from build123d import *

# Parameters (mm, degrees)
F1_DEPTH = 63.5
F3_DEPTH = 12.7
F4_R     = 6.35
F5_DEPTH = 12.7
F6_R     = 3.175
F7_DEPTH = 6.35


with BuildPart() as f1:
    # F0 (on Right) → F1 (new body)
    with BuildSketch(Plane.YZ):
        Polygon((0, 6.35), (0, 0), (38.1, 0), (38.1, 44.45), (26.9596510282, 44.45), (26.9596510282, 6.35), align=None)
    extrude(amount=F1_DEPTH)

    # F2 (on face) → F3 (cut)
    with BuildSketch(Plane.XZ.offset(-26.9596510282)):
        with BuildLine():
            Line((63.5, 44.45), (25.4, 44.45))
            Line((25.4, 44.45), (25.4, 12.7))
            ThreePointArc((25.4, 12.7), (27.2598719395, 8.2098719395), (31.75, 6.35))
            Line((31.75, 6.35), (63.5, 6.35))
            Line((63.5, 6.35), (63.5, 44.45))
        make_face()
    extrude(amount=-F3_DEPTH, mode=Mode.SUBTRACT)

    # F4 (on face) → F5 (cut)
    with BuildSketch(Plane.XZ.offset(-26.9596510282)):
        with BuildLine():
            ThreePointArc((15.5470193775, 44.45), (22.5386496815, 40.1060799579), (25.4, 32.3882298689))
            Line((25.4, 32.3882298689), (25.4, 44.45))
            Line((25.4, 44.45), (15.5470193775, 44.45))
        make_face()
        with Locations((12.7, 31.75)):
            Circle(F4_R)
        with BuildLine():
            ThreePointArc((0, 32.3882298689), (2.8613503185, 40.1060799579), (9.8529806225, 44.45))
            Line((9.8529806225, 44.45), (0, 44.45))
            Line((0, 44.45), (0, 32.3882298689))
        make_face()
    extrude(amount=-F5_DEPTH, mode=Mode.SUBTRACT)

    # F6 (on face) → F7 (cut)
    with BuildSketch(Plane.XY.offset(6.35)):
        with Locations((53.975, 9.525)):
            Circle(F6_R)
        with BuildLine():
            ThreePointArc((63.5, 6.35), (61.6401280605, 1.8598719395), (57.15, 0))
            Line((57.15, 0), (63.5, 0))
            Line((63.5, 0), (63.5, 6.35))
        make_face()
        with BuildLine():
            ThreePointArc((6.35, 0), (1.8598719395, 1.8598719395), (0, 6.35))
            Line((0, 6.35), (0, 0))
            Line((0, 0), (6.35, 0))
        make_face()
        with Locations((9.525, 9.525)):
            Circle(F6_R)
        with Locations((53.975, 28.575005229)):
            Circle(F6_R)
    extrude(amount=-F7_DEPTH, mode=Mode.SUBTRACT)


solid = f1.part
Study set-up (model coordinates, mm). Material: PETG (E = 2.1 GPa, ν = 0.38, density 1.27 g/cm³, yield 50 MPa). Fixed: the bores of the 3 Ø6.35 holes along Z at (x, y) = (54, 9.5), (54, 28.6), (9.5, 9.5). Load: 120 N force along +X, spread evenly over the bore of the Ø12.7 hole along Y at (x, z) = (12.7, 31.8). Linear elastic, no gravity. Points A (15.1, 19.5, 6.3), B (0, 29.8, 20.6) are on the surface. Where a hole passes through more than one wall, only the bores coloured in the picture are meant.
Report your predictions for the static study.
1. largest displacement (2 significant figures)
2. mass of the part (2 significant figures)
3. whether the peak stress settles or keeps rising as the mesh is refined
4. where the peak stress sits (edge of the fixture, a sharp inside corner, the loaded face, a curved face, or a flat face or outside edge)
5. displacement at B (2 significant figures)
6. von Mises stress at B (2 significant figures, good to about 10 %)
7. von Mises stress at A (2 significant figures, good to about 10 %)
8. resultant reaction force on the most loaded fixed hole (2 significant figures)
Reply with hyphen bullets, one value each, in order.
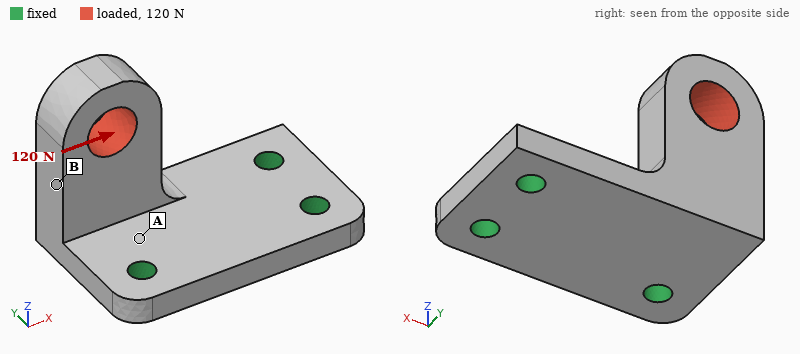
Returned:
- 0.58 mm
- 30 g
- keeps rising
- edge of the fixture
- 0.34 mm
- 1.8 MPa
- 5.1 MPa
- 92 N
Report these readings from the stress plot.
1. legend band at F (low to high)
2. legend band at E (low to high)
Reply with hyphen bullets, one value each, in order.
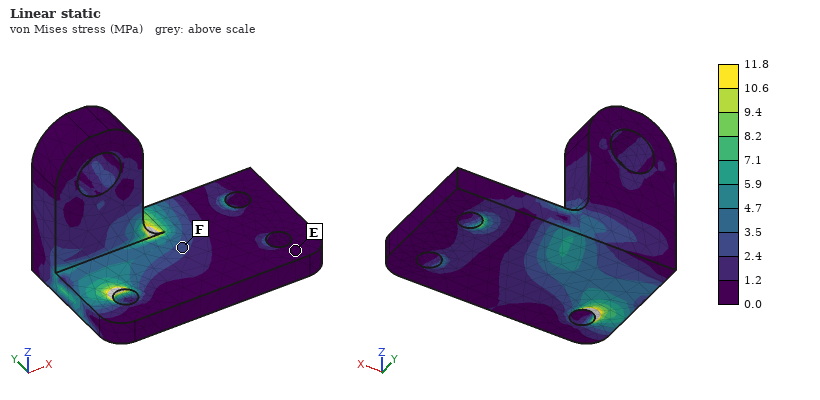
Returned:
- 2.4 to 3.5 MPa
- 0.0 to 1.2 MPa
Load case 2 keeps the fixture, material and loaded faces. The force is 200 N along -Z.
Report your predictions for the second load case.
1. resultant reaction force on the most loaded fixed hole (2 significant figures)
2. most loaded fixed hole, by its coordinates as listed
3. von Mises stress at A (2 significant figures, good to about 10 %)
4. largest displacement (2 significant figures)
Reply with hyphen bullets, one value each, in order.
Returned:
- 160 N
- (9.5, 9.5)
- 7.1 MPa
- 0.98 mm
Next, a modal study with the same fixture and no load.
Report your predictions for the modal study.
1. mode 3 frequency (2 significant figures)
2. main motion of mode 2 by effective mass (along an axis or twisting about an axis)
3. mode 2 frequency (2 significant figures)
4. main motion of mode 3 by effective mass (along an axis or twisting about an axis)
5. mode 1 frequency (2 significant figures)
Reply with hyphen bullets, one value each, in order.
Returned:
- 1800 Hz
- along X
- 1100 Hz
- along Z
- 580 Hz
